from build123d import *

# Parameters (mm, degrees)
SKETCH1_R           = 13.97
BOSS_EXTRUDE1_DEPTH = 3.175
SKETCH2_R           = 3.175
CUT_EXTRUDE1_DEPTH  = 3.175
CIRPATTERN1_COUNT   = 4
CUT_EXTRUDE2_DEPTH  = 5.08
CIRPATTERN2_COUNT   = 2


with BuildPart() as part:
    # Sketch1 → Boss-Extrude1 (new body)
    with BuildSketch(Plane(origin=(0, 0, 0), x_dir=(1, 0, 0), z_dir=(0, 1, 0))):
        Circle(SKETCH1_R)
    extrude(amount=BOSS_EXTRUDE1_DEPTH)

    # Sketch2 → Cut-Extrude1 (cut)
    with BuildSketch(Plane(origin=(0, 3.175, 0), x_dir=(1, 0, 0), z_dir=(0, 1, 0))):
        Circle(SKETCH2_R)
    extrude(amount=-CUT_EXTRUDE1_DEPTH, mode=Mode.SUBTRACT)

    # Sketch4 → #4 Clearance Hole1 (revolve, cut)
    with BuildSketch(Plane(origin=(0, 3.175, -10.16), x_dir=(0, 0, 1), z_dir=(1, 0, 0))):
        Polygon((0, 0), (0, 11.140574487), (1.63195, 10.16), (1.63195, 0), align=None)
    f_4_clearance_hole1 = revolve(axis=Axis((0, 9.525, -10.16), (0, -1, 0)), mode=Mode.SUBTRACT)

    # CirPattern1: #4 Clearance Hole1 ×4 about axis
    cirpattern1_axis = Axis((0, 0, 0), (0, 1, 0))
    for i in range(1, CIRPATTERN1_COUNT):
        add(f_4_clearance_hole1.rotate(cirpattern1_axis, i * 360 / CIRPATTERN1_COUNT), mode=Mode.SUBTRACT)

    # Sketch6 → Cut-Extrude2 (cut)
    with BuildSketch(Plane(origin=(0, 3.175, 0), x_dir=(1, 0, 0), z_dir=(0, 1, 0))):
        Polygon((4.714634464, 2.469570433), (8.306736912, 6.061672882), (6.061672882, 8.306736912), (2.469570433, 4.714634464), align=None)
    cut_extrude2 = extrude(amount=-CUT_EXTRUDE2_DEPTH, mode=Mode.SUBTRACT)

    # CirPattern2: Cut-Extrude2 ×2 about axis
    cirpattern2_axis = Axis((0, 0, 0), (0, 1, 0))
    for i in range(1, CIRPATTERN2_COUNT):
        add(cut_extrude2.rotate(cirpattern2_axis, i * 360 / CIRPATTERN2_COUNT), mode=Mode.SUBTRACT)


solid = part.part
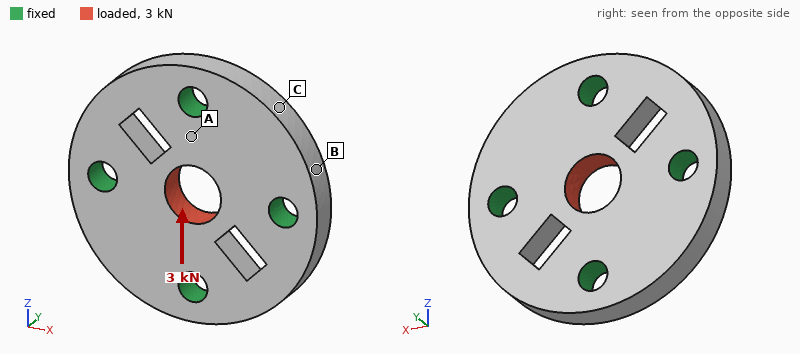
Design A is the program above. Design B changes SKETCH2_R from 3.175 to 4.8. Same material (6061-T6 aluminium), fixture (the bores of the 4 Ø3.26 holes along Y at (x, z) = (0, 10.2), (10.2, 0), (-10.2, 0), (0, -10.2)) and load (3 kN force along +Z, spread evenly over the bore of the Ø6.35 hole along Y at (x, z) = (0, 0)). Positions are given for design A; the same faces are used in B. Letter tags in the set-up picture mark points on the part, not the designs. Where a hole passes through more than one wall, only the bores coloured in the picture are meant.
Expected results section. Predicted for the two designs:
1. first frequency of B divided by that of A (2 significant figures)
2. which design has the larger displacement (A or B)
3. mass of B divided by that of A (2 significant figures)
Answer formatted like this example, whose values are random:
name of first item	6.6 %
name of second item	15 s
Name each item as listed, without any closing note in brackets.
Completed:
first frequency of B divided by that of A	1.0
which design has the larger displacement	B
mass of B divided by that of A	0.92
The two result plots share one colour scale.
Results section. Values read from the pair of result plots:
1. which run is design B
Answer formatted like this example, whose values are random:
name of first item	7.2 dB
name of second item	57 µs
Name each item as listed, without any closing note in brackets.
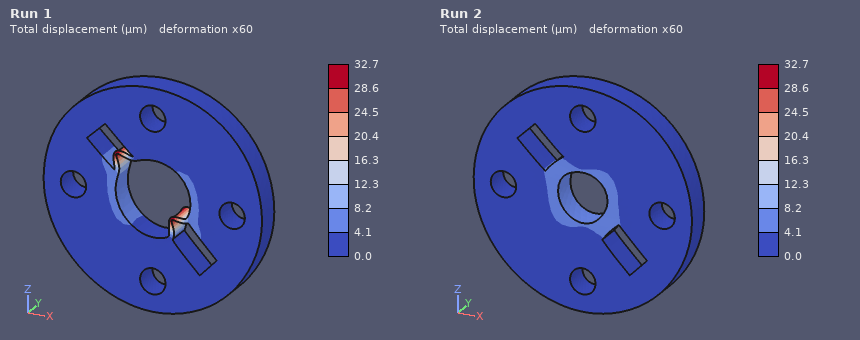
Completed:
which run is design B	Run 1
